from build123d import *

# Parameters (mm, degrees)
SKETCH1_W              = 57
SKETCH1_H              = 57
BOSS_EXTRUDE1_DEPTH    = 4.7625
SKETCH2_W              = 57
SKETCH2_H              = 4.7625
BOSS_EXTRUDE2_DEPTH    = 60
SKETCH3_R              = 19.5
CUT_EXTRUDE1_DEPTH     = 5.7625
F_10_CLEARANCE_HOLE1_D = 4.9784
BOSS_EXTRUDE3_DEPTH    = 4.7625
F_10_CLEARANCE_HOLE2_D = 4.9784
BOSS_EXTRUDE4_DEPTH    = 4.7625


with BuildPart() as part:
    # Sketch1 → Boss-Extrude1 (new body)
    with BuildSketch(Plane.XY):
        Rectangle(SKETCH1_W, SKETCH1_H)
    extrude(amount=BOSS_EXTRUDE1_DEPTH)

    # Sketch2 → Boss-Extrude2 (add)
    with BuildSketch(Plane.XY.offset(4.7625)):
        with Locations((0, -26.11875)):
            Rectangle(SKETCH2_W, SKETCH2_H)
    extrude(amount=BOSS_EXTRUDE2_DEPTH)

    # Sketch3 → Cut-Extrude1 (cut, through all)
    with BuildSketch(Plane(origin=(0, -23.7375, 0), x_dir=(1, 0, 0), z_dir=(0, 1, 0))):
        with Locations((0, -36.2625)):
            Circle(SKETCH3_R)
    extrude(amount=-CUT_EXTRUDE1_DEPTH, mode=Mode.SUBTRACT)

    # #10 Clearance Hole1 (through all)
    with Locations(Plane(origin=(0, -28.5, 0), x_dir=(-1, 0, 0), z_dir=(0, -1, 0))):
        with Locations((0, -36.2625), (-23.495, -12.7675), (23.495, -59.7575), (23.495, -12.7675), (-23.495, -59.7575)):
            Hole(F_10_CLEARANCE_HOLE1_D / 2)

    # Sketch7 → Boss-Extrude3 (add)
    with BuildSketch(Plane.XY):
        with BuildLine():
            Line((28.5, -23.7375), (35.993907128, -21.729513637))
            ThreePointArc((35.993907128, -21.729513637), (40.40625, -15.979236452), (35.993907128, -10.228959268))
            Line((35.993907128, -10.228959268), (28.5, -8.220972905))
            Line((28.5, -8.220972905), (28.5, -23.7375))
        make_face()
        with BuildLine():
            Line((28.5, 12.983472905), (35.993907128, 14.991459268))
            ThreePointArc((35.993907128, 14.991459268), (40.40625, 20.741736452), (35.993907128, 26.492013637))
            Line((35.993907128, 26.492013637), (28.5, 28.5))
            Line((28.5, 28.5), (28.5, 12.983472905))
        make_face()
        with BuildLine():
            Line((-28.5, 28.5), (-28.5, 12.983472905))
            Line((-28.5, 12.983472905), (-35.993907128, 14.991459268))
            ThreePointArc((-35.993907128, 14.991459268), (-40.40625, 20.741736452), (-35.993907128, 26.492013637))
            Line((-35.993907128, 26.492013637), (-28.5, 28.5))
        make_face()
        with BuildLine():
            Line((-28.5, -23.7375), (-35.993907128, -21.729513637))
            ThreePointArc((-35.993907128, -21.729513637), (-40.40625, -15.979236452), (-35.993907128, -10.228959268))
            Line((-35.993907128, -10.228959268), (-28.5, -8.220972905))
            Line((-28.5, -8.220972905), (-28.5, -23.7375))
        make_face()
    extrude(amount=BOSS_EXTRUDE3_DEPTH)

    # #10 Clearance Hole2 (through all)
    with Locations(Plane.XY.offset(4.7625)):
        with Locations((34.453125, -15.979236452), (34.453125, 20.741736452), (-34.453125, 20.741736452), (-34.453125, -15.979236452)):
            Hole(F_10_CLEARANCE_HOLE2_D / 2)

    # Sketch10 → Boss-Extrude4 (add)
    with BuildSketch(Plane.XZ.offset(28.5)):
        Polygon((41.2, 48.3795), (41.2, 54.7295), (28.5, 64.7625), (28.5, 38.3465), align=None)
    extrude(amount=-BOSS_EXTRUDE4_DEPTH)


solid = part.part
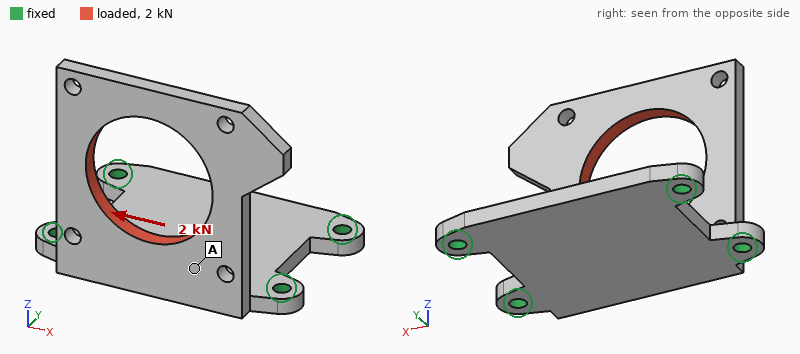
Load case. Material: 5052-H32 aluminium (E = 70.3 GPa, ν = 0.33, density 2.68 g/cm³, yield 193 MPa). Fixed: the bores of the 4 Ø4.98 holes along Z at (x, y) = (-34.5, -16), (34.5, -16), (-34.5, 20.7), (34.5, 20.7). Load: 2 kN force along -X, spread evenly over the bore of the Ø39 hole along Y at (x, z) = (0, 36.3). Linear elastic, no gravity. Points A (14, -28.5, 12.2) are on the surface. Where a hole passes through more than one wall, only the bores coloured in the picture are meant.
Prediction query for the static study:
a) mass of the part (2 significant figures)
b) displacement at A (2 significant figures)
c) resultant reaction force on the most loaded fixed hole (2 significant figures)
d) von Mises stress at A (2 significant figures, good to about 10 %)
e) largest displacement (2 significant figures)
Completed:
78 g
0.044 mm
1.5 kN
26 MPa
0.28 mm
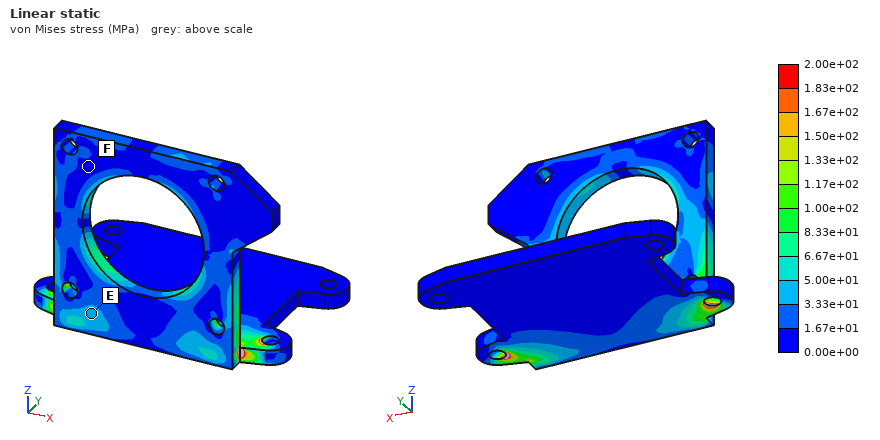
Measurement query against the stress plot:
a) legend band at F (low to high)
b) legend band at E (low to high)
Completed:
0.00e+00 to 1.67e+01 MPa
3.33e+01 to 5.00e+01 MPa
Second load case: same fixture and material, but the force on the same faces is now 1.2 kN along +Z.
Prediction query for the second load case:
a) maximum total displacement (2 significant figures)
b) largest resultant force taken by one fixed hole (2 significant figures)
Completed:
0.20 mm
690 N
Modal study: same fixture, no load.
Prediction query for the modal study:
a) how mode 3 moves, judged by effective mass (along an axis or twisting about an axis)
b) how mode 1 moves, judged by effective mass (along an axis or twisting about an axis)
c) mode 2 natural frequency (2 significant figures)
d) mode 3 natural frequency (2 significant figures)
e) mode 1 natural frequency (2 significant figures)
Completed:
along X
along Y
1600 Hz
2900 Hz
700 Hz
